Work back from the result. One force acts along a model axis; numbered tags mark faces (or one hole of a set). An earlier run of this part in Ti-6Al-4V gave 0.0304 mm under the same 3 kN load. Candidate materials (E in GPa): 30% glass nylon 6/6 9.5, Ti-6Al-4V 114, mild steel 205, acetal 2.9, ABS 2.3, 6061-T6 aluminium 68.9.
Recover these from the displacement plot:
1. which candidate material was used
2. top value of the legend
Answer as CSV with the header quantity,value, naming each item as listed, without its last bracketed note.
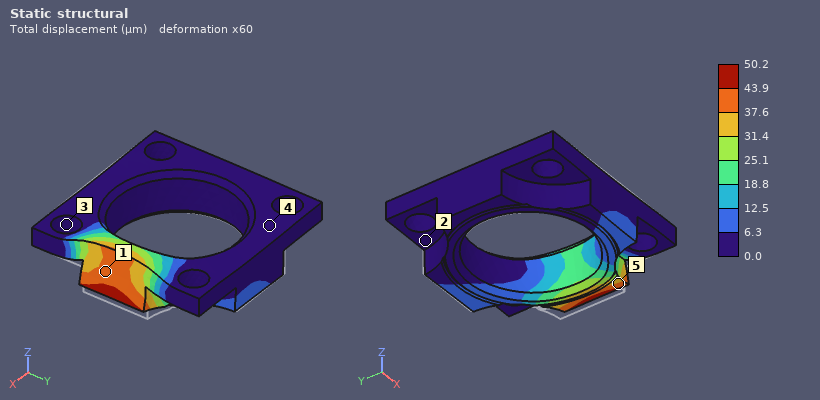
quantity,value
which candidate material was used,6061-T6 aluminium
top value of the legend,50.2 µm
